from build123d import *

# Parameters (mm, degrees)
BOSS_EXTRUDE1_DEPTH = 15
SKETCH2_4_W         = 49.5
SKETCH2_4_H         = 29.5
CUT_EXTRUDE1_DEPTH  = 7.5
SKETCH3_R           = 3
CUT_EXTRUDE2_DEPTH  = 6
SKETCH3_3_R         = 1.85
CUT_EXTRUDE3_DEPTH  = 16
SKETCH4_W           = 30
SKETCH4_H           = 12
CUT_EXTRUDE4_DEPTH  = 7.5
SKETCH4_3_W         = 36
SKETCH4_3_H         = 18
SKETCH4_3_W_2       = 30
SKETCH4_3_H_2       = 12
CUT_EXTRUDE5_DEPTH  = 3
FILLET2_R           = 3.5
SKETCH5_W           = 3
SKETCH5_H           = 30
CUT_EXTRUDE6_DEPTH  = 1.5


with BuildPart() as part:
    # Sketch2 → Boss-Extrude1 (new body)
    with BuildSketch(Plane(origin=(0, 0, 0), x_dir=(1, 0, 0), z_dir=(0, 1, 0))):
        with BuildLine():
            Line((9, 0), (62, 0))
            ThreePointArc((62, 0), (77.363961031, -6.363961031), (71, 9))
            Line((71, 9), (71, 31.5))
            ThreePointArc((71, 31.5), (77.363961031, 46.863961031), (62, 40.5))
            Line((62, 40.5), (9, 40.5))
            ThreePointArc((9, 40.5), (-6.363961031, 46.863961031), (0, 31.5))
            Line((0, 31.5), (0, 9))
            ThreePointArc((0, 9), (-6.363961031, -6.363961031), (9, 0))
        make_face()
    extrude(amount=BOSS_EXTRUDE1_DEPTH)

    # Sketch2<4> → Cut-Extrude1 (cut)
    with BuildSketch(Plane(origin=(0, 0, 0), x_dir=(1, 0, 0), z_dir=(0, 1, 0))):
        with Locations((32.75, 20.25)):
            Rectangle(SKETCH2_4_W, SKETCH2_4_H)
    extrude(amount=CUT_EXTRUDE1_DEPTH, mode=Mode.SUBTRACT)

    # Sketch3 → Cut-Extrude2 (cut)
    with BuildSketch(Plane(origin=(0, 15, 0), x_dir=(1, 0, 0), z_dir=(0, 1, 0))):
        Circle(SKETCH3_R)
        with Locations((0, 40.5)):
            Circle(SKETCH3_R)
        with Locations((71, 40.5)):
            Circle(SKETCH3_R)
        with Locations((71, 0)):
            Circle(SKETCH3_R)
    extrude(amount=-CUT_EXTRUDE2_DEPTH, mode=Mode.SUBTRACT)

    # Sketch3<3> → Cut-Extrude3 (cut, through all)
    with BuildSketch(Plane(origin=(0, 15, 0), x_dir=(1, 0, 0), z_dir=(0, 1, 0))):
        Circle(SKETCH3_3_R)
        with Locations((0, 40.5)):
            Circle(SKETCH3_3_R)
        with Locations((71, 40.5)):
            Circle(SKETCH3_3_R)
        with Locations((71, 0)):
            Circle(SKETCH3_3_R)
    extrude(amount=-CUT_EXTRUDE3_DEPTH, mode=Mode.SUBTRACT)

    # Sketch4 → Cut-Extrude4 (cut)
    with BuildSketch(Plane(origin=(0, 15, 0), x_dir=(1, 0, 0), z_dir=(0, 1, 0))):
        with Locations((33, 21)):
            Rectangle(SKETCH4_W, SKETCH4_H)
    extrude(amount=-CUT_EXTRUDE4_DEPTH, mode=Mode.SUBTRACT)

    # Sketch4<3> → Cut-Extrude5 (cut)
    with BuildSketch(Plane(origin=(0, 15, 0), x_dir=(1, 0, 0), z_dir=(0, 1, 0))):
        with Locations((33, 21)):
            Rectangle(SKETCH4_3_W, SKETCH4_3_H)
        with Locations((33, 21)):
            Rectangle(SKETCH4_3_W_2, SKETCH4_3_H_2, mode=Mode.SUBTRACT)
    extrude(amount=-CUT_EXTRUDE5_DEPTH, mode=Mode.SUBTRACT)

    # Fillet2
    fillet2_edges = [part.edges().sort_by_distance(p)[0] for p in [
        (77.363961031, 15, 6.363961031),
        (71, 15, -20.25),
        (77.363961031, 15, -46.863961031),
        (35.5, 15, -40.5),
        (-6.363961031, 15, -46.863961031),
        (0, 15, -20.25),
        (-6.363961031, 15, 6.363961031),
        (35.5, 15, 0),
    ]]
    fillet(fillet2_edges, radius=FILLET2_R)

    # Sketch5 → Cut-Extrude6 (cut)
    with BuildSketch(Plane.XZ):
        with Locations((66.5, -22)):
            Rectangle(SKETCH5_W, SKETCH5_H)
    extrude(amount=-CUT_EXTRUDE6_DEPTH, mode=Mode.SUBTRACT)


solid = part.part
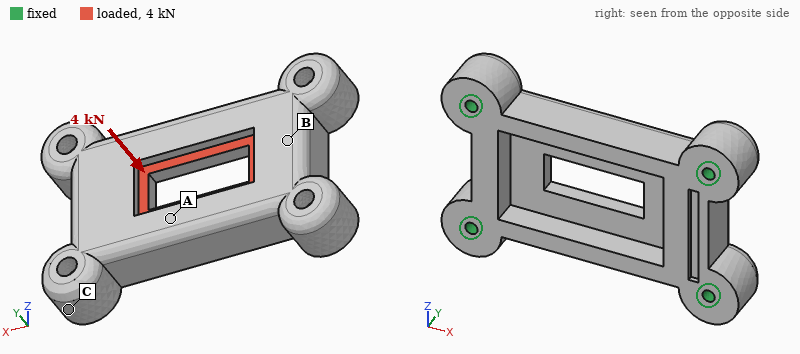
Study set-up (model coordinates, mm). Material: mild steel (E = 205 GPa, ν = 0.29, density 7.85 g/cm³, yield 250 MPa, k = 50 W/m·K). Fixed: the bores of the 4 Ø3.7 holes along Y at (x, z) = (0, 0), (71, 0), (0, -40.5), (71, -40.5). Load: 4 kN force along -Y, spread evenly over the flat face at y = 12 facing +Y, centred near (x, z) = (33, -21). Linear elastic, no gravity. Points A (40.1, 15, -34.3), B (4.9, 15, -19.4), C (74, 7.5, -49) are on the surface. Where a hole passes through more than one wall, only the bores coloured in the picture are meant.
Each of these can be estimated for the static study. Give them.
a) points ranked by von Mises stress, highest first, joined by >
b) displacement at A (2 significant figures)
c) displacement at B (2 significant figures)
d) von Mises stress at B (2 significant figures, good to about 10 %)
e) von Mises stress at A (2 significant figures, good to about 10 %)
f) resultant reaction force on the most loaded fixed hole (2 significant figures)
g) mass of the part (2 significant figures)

A > B > C
12 µm
4.8 µm
24 MPa
48 MPa
1.6 kN
300 g
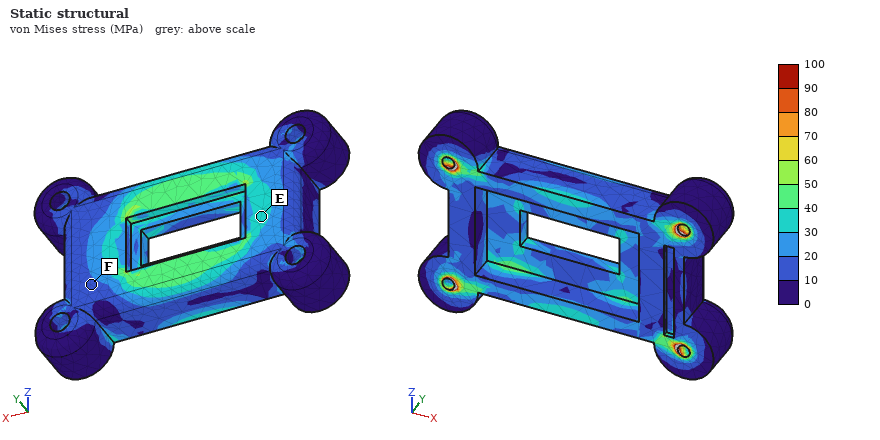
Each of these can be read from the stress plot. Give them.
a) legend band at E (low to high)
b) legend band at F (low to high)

30 to 40 MPa
10 to 20 MPa
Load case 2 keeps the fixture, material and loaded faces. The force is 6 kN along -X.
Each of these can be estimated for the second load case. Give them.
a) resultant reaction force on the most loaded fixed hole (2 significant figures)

1.7 kN
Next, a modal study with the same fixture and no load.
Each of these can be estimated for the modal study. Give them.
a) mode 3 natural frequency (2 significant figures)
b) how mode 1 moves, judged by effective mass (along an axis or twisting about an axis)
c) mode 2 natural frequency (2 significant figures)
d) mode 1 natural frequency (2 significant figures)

17 kHz
along Y
12 kHz
9700 Hz
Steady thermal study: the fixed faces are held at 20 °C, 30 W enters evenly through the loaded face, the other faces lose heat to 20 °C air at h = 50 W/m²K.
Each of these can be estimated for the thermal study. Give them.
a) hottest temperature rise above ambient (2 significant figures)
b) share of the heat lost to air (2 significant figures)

28 K
20 %
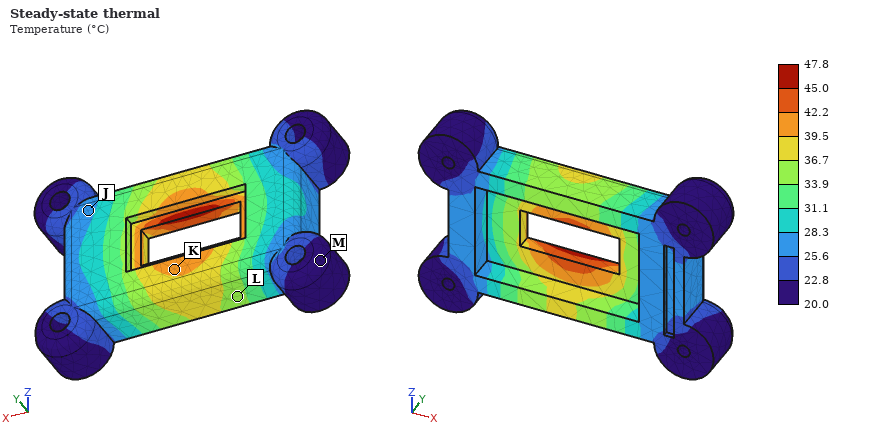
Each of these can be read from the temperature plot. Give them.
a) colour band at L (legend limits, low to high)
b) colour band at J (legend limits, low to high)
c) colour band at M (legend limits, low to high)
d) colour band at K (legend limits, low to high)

33.9 to 36.7 °C
25.6 to 28.3 °C
20.0 to 22.8 °C
39.5 to 42.2 °C
